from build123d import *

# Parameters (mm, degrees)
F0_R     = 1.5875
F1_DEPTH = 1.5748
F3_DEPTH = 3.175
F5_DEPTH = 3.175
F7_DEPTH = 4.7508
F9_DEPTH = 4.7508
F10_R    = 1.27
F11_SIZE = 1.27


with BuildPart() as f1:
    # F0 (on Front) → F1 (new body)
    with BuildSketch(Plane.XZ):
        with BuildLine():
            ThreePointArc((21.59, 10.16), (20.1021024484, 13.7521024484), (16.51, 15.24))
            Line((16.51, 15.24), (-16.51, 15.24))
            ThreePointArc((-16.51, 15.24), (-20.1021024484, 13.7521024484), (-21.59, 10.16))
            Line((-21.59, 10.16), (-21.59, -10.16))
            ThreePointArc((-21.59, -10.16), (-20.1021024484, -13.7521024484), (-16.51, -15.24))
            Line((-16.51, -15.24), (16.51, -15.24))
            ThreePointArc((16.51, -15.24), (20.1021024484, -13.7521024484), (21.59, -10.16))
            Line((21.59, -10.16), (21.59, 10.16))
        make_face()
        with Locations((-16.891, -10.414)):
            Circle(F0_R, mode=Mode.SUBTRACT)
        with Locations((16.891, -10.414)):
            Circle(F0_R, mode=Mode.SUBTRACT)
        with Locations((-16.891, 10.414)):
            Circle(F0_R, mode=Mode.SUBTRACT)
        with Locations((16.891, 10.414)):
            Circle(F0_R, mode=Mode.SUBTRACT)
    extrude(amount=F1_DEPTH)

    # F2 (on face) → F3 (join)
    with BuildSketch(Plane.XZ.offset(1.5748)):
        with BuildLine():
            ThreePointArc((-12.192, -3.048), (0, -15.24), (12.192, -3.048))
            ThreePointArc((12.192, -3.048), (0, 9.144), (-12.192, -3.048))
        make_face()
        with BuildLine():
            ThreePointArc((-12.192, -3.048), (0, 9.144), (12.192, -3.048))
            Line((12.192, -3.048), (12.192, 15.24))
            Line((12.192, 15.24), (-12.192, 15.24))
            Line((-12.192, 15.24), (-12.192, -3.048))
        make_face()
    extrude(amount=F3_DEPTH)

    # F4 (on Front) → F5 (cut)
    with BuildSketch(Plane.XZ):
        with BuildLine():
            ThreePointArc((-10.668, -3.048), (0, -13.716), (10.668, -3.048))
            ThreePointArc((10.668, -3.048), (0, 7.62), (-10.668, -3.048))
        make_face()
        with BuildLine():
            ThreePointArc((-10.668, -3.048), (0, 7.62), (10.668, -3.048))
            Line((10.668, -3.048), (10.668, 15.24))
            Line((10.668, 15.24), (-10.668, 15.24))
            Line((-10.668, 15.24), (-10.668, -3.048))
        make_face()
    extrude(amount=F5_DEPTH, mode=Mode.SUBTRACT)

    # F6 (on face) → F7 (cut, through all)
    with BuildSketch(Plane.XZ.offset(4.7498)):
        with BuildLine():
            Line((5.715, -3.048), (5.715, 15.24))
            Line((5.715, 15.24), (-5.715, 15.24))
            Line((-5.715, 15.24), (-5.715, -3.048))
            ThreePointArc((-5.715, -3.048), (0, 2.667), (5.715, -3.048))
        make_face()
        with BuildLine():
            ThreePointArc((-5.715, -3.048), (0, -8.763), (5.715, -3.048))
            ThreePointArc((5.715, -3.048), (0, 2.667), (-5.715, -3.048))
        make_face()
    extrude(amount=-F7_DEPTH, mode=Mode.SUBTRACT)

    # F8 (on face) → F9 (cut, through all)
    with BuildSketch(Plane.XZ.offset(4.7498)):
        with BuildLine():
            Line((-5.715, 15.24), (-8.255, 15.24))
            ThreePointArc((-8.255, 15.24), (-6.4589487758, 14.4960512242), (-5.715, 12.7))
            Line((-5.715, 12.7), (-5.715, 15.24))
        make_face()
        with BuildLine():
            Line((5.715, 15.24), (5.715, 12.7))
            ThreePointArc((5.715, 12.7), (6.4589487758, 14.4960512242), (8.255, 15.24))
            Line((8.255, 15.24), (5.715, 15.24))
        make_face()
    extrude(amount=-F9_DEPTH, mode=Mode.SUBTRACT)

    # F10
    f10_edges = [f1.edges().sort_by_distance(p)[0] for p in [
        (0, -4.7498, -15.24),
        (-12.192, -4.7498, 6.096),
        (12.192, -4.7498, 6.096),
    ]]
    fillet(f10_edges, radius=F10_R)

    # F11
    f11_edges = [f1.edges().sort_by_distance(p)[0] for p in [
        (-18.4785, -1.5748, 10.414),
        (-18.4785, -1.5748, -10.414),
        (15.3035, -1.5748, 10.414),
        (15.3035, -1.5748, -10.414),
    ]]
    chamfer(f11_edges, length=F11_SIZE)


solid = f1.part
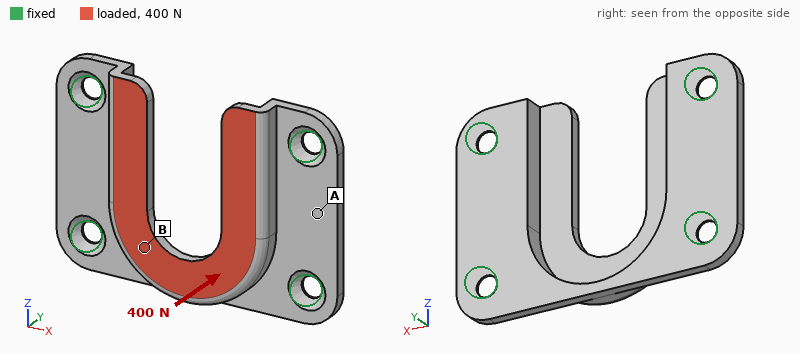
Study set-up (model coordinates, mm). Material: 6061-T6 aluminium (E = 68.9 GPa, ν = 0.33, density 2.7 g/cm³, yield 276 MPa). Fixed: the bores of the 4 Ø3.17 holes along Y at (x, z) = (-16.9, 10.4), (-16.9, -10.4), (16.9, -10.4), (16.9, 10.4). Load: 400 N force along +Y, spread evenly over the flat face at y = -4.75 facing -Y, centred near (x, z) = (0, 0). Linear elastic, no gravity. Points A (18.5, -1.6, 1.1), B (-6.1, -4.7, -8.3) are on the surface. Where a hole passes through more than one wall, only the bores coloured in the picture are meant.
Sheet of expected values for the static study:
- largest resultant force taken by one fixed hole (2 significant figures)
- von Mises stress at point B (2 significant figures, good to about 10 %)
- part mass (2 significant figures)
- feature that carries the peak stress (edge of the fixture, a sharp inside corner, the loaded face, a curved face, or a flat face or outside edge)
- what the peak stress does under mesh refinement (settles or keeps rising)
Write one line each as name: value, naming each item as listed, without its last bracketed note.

largest resultant force taken by one fixed hole: 240 N
von Mises stress at point B: 65 MPa
part mass: 5.0 g
feature that carries the peak stress: edge of the fixture
what the peak stress does under mesh refinement: keeps rising
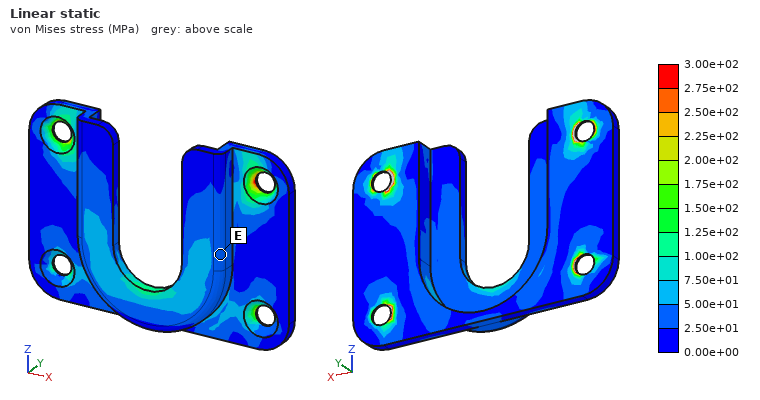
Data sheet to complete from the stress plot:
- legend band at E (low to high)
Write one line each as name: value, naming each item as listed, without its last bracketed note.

legend band at E: 2.50e+01 to 5.00e+01 MPa
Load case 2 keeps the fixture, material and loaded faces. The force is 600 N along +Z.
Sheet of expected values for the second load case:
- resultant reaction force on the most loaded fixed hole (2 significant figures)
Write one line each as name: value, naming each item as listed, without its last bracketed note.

resultant reaction force on the most loaded fixed hole: 200 N
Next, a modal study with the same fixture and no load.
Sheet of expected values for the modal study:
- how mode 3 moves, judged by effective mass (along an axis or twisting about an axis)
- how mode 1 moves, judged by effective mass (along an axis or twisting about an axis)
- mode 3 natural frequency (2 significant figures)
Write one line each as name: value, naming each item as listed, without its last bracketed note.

how mode 3 moves, judged by effective mass: along Y
how mode 1 moves, judged by effective mass: along Y
mode 3 natural frequency: 11 kHz
